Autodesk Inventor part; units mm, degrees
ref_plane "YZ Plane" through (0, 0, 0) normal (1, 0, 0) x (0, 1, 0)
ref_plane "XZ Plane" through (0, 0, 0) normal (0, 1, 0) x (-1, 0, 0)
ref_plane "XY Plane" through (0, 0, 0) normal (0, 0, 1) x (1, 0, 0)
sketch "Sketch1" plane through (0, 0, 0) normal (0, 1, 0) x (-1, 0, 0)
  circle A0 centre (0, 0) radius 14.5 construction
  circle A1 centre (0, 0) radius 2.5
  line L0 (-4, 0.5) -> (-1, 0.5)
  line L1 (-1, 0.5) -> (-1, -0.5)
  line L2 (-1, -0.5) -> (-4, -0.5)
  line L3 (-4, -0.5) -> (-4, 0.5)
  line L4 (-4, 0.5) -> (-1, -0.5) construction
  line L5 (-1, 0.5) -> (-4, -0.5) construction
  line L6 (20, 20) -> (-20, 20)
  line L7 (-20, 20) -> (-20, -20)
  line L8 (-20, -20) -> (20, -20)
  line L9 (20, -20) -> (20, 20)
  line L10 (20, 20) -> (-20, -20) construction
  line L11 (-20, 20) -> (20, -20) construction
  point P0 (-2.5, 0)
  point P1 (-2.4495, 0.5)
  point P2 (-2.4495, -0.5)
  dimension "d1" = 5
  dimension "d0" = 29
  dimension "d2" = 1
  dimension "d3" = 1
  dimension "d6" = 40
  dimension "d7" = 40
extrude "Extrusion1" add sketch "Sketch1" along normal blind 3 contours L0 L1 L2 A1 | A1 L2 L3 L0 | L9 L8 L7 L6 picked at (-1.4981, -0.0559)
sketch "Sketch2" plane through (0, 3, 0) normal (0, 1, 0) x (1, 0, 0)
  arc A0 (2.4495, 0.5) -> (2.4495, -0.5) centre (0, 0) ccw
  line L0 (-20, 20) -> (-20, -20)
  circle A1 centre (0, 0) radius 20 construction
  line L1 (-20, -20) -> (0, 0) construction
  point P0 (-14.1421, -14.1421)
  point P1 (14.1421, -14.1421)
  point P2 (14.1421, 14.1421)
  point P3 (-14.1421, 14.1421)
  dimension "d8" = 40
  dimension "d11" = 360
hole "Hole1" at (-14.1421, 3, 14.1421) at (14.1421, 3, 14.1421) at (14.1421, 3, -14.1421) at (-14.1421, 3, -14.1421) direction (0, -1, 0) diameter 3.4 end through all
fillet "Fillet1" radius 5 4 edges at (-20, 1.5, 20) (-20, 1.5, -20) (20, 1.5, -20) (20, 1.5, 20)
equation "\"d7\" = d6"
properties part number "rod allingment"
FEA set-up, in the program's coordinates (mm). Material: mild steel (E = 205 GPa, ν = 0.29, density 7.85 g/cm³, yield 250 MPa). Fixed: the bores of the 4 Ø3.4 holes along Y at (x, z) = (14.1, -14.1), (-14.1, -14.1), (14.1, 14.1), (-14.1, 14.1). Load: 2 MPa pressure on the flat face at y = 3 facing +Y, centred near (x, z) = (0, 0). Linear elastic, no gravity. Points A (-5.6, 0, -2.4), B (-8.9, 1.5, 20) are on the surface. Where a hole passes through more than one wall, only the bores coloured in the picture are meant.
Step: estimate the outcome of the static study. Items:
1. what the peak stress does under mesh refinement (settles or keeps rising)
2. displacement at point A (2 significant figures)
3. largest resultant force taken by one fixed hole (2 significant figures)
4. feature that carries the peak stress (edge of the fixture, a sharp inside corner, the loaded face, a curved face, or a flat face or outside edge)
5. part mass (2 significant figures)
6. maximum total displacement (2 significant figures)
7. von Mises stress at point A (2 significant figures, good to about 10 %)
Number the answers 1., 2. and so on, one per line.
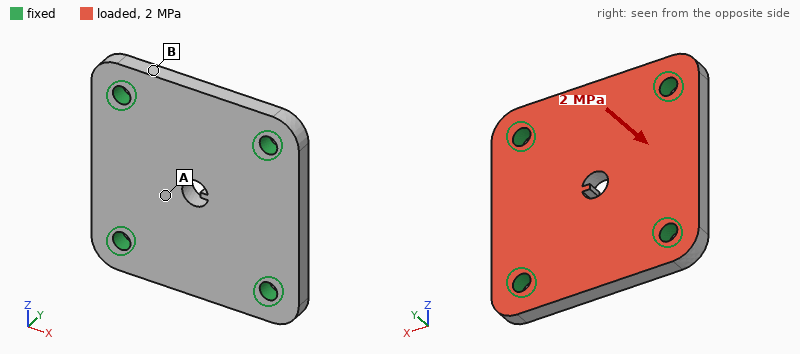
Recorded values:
1. keeps rising
2. 14 µm
3. 760 N
4. edge of the fixture
5. 36 g
6. 18 µm
7. 40 MPa
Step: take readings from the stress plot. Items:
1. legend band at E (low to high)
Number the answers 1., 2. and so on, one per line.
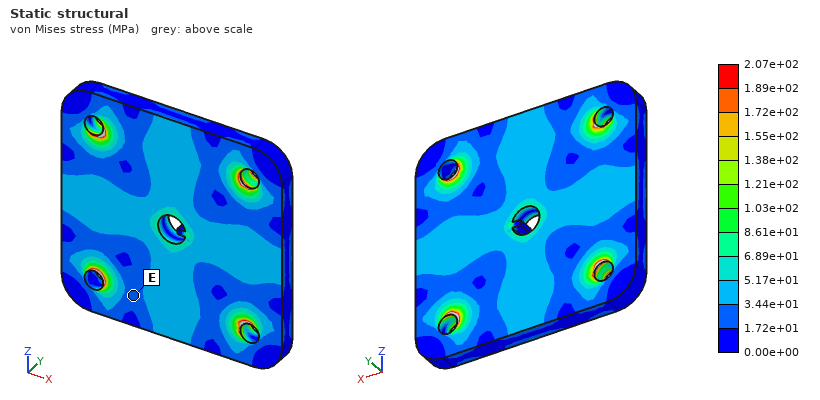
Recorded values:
1. 1.72e+01 to 3.44e+01 MPa
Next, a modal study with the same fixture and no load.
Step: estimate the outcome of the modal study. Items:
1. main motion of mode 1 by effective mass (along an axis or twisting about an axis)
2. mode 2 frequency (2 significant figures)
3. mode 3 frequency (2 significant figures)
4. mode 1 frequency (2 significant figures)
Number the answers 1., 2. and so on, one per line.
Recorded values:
1. along Y
2. 21 kHz
3. 21 kHz
4. 14 kHz
